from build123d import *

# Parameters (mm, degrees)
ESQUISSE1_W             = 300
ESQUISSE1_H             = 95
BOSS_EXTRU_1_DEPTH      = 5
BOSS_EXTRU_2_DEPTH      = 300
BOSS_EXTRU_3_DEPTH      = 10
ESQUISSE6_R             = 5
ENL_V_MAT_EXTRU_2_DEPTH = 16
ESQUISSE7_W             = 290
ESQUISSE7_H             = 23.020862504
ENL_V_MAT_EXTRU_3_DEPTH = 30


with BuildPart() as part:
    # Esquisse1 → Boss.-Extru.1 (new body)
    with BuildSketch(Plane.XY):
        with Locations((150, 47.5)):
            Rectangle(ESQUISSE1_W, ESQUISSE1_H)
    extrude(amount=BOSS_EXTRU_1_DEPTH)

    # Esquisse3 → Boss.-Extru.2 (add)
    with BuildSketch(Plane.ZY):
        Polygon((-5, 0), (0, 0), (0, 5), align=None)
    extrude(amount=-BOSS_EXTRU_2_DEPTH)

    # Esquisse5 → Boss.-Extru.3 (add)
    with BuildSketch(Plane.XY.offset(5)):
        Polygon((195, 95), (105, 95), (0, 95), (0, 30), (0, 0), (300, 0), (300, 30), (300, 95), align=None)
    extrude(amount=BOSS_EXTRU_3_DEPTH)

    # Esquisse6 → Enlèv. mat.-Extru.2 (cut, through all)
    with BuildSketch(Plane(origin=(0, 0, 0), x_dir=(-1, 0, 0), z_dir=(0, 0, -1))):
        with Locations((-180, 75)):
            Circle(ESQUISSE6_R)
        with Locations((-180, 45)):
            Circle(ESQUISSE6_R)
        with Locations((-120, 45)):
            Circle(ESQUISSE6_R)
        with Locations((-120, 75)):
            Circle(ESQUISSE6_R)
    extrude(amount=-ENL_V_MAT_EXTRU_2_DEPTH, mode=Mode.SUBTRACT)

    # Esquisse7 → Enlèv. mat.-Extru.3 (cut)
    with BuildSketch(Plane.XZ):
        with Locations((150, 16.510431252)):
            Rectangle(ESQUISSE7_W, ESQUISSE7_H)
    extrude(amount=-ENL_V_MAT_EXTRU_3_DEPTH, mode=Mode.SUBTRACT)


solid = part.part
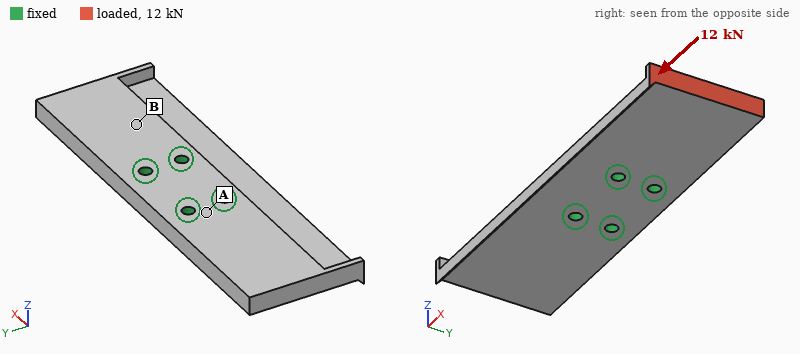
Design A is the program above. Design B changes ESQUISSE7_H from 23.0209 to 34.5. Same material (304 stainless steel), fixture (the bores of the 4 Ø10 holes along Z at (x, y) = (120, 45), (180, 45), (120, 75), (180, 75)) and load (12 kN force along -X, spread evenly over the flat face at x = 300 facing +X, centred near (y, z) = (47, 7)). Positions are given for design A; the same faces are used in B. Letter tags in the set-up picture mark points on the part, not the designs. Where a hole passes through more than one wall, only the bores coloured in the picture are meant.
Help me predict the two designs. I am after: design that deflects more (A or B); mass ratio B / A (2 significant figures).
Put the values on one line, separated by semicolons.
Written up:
B; 0.87
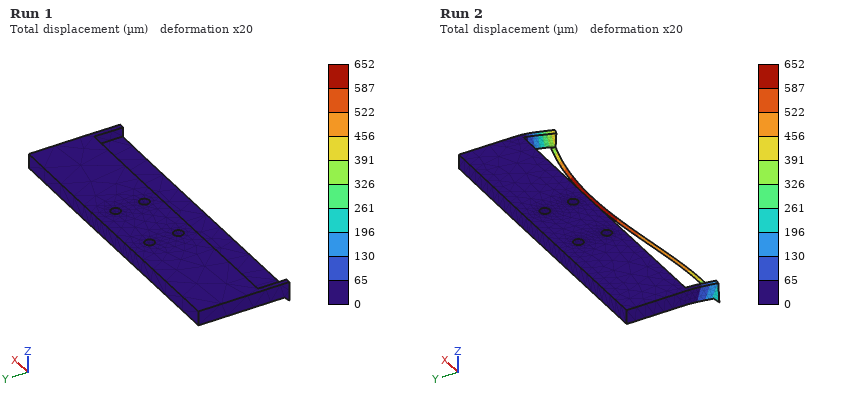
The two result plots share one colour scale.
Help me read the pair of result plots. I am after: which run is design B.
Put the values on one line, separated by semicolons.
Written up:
Run 2
